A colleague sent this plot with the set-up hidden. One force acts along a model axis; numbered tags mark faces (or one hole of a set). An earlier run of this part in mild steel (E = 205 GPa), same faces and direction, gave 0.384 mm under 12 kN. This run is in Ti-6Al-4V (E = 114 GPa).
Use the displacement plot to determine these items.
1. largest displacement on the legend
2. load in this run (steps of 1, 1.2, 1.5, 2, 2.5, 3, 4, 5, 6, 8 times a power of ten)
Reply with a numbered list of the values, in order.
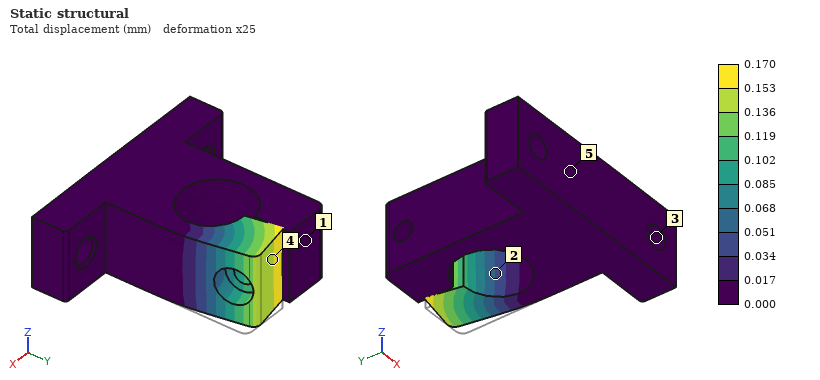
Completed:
1. 0.170 mm
2. 3 kN
